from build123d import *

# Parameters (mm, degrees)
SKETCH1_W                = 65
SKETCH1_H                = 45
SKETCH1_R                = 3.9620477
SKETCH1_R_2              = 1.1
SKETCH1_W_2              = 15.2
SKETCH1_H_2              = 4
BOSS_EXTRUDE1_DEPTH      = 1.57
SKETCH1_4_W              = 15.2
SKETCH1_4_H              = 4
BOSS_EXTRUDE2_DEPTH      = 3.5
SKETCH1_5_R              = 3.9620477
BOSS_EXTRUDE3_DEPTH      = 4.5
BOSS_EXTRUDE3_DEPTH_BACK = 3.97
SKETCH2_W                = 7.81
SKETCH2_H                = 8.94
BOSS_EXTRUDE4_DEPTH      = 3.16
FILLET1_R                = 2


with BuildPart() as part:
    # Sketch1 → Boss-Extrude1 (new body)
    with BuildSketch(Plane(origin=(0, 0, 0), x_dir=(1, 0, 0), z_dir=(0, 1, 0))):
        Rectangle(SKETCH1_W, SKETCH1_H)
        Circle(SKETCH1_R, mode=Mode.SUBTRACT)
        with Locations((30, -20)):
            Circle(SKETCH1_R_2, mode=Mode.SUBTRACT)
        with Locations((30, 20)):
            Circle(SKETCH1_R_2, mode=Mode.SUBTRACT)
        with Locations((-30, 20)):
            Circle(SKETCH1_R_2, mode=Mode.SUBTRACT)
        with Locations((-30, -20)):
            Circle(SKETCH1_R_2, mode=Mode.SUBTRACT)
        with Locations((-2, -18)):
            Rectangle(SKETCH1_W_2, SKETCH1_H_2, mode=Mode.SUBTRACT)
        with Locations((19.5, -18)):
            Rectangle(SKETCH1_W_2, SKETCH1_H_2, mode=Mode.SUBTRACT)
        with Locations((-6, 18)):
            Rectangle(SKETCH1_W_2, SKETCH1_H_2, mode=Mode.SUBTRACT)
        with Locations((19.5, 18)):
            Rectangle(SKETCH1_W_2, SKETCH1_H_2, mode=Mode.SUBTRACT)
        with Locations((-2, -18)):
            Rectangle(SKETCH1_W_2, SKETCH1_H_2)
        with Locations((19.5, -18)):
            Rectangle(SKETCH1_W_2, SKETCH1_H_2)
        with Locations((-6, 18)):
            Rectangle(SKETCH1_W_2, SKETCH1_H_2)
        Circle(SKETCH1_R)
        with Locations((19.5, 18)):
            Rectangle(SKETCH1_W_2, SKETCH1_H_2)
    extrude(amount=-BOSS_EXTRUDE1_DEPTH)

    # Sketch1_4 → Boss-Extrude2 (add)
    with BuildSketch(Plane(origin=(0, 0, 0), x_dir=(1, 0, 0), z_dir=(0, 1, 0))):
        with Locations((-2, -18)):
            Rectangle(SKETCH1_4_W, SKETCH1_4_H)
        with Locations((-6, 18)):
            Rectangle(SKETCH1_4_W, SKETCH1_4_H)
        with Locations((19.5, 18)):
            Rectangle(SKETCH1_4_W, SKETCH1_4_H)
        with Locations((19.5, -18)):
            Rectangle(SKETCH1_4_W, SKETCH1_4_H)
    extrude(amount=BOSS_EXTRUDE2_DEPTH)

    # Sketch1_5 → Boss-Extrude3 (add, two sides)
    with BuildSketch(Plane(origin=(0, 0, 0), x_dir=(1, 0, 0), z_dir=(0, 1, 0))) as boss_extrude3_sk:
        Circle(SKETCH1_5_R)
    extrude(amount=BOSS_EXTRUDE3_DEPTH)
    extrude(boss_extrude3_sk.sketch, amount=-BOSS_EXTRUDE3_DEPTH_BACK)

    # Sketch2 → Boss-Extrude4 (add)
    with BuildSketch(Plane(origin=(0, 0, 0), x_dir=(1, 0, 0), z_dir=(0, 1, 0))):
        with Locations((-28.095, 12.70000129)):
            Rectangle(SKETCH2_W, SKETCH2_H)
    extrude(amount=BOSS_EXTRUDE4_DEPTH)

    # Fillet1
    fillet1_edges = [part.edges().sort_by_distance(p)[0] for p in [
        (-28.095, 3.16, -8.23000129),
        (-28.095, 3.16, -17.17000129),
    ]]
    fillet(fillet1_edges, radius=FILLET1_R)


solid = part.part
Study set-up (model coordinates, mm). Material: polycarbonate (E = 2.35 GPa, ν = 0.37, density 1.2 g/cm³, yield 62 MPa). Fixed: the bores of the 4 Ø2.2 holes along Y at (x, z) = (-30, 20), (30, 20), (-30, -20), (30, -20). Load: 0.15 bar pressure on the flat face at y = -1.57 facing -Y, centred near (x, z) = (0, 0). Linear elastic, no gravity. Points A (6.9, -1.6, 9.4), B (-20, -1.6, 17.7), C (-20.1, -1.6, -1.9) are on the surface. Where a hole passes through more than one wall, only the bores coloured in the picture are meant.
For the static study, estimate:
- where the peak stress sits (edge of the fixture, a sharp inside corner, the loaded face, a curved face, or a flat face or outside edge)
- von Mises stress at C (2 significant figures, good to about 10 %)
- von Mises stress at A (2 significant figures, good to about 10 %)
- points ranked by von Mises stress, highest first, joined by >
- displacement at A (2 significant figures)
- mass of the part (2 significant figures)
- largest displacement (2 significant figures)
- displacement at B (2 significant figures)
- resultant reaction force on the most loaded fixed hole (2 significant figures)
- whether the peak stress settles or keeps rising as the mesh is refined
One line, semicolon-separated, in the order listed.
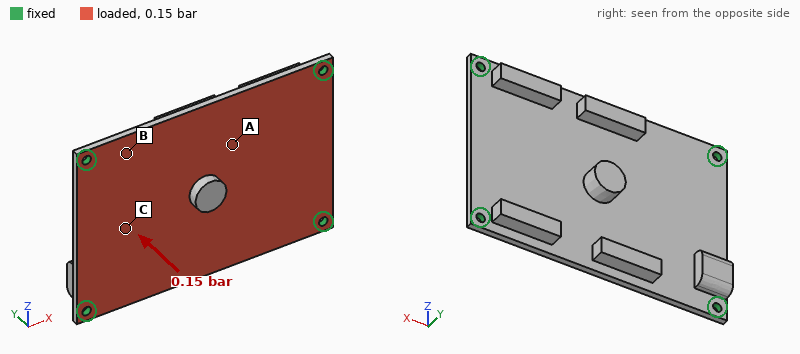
edge of the fixture; 3.1 MPa; 5.3 MPa; A > C > B; 0.70 mm; 7.2 g; 0.75 mm; 0.28 mm; 11 N; keeps rising
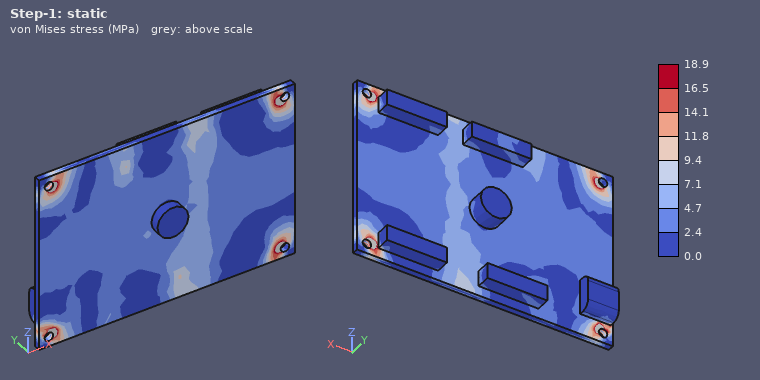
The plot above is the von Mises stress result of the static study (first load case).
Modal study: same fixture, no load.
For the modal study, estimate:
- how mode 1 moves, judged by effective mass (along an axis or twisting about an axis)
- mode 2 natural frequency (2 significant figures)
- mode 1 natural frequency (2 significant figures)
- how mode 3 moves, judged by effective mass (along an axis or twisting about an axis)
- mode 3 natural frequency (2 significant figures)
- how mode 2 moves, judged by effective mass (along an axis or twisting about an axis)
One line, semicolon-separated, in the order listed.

along Y; 840 Hz; 510 Hz; twisting about Z; 1300 Hz; twisting about X
